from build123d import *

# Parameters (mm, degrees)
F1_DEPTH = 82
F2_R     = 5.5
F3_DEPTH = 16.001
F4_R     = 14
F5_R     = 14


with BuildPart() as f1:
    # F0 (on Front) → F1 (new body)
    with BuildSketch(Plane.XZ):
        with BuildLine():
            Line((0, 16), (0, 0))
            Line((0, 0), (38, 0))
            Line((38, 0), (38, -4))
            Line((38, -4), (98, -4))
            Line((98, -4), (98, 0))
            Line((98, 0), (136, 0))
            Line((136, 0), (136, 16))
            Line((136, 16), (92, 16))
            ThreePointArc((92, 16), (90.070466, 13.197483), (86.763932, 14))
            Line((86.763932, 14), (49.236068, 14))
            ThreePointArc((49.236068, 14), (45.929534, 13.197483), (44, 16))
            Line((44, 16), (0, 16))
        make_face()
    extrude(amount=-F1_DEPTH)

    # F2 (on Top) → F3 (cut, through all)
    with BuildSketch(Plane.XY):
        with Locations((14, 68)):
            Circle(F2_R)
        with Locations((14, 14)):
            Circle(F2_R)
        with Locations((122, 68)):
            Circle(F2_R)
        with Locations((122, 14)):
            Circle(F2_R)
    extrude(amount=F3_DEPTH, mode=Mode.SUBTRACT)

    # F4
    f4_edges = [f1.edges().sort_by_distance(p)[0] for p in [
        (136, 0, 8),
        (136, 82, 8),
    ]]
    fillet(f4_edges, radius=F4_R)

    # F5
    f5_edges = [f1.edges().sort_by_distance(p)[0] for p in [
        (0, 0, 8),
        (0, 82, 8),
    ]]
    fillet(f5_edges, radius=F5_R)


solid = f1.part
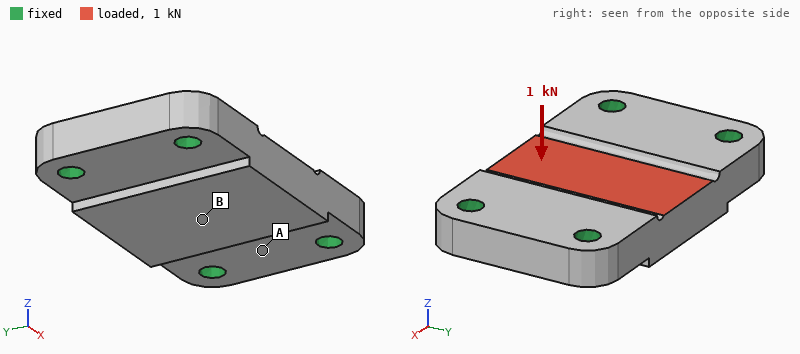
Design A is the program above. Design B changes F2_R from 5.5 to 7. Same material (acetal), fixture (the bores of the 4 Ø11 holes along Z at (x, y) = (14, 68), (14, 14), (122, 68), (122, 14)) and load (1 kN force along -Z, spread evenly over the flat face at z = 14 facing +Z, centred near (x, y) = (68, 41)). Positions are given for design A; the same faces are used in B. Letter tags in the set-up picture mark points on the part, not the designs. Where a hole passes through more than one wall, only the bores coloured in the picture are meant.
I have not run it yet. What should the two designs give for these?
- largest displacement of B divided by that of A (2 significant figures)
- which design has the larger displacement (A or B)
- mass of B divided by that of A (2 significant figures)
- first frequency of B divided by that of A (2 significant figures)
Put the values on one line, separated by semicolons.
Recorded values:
0.89; A; 0.98; 1.1
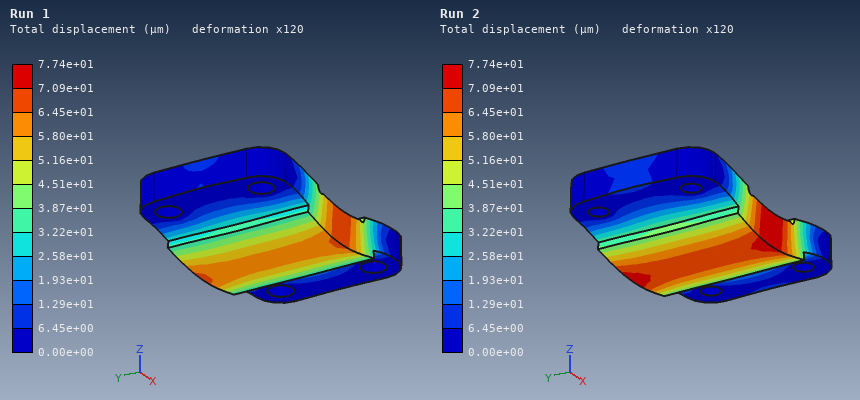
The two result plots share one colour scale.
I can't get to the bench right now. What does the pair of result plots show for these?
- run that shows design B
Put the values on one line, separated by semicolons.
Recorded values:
Run 1
